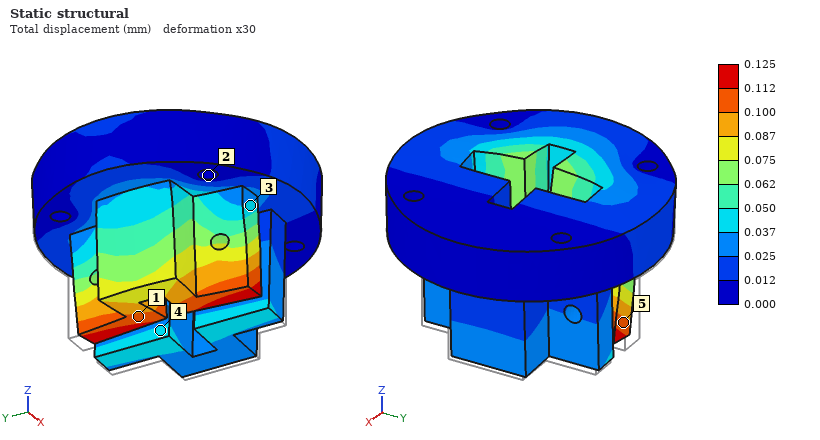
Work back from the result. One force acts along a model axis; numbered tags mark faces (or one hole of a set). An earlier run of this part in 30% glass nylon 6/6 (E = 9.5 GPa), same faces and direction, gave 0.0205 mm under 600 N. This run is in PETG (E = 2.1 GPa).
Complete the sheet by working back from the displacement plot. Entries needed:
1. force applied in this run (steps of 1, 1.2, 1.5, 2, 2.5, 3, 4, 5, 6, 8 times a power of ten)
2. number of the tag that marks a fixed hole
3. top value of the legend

800 N
2
0.125 mm
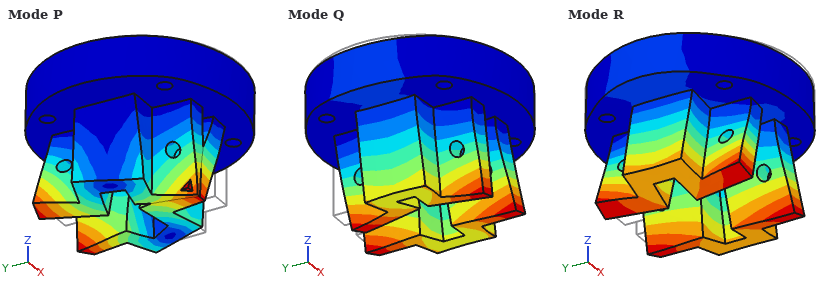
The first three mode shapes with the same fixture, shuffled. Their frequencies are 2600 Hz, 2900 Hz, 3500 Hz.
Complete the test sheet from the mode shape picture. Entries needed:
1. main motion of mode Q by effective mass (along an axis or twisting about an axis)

along X
